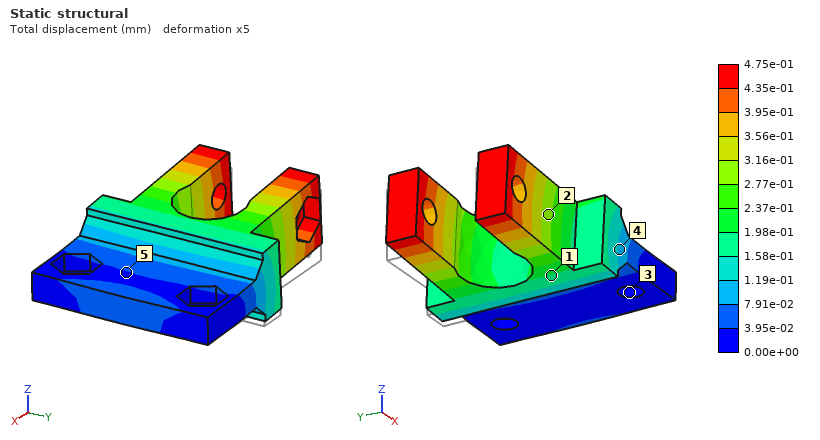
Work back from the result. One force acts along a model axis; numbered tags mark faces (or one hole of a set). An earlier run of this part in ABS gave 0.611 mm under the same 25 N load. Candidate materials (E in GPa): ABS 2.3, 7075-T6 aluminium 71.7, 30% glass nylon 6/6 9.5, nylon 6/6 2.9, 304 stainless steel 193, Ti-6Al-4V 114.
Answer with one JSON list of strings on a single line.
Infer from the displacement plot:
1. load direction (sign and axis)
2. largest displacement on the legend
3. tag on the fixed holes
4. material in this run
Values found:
["+Z", "4.75e-01 mm", "3", "nylon 6/6"]
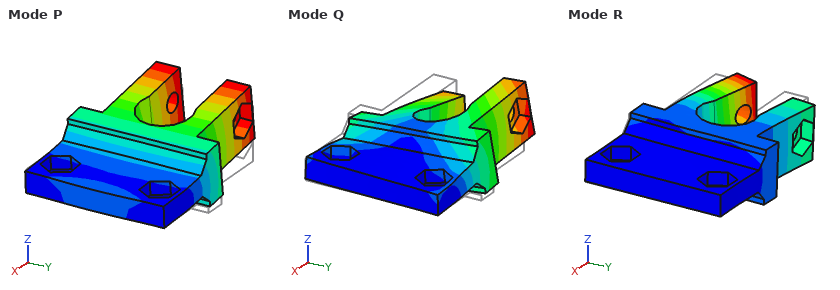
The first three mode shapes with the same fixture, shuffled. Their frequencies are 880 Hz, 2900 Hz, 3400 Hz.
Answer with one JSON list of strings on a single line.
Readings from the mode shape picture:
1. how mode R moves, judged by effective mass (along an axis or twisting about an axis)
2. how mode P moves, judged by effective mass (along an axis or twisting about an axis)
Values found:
["along Y", "along Z"]
